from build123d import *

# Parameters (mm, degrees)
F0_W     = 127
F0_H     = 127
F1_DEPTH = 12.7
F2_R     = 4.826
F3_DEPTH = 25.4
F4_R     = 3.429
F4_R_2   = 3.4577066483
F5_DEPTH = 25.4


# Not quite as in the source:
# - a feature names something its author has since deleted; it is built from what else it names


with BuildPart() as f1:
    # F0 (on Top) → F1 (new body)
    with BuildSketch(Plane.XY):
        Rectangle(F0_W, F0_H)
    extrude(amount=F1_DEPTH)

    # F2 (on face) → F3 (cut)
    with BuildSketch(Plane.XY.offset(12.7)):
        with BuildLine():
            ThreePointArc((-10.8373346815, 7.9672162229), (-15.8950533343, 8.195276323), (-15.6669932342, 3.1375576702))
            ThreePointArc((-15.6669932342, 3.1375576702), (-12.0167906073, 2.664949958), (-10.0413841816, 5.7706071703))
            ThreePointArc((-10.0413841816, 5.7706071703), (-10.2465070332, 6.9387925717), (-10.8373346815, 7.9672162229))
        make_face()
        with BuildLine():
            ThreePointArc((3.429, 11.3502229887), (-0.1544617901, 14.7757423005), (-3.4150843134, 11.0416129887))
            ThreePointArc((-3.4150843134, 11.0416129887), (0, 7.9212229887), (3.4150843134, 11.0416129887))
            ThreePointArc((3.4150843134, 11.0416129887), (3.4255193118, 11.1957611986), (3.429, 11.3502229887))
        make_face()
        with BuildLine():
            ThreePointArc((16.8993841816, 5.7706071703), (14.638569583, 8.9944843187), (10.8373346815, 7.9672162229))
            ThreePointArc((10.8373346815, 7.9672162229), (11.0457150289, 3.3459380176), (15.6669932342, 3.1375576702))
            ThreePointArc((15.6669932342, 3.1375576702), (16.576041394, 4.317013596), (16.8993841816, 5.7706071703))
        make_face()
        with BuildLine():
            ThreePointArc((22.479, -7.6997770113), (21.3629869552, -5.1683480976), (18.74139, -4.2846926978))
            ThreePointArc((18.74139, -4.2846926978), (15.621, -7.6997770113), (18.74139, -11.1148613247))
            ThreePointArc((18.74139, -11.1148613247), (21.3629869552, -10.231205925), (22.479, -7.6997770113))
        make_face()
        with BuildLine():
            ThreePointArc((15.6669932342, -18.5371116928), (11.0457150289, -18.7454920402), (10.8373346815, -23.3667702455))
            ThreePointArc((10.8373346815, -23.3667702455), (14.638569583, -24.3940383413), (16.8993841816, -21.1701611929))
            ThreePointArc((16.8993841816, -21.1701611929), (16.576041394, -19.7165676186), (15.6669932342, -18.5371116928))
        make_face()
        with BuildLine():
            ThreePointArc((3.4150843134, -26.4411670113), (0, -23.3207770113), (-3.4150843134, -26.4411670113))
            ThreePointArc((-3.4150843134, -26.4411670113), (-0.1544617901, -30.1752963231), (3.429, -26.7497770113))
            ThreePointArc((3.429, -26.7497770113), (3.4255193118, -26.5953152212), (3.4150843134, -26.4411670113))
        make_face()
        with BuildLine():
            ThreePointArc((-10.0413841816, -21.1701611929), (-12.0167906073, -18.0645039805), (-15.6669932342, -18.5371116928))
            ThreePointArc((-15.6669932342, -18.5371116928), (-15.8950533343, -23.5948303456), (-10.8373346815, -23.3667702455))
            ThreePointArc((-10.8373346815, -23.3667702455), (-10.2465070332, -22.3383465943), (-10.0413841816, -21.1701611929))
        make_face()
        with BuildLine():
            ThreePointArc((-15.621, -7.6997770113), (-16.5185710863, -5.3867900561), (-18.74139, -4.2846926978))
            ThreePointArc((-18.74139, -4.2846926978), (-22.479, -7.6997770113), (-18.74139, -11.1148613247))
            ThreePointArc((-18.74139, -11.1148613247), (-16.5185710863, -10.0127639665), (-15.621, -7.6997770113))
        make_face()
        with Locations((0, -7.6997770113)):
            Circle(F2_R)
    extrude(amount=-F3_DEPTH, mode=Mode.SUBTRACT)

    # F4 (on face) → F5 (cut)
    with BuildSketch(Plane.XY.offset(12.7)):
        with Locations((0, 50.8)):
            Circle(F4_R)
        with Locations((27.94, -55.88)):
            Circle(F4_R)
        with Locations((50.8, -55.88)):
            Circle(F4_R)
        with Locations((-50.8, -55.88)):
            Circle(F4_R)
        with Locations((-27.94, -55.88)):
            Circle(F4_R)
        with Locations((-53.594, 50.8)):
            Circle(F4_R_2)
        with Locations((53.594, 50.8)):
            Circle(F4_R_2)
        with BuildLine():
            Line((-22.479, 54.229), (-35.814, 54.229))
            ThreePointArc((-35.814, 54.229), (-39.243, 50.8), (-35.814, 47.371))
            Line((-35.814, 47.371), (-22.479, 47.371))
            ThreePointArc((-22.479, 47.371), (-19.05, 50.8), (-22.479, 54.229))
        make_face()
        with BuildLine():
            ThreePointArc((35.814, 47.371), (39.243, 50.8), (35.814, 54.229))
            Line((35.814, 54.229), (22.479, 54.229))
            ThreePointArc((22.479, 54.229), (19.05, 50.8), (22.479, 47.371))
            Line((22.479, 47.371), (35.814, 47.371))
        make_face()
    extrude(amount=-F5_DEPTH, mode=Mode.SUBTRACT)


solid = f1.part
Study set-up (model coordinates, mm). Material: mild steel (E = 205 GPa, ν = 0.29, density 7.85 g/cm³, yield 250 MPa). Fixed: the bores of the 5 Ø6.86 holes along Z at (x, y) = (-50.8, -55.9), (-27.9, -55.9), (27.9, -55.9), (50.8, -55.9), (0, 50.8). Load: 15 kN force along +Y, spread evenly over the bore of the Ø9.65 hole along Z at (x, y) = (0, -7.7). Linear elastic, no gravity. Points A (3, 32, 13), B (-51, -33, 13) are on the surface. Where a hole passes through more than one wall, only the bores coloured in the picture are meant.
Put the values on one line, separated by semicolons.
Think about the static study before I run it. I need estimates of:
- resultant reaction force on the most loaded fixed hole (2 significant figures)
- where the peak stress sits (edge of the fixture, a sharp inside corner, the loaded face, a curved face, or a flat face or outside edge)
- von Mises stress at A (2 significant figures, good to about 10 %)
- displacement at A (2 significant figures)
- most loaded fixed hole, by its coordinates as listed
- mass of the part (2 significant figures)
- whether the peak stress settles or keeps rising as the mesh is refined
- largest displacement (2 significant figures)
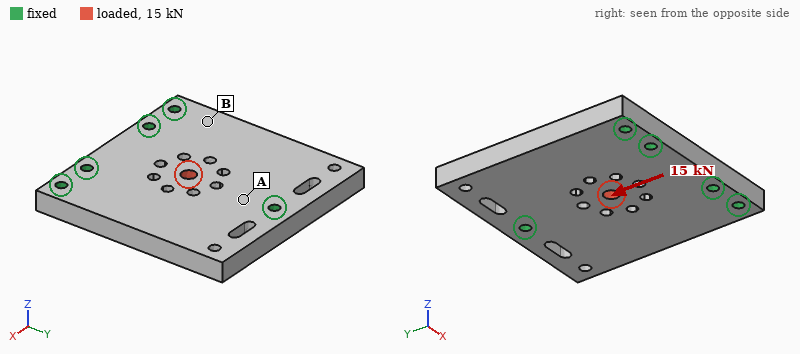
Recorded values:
4.7 kN; a sharp inside corner; 14 MPa; 1.3 µm; (0, 50.8); 1.5 kg; keeps rising; 5.4 µm
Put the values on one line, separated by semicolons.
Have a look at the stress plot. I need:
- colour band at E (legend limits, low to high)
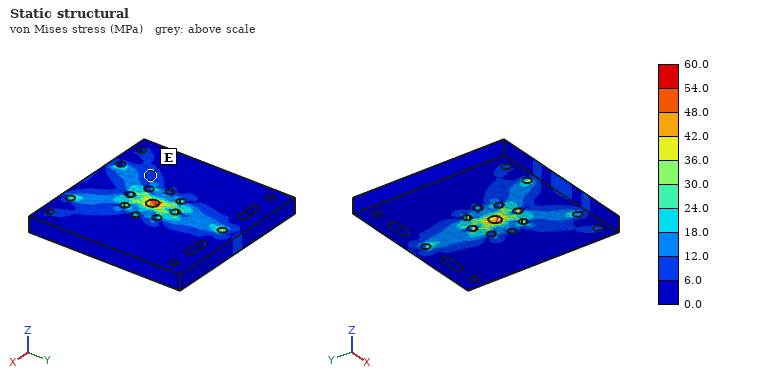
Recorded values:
6.0 to 12.0 MPa
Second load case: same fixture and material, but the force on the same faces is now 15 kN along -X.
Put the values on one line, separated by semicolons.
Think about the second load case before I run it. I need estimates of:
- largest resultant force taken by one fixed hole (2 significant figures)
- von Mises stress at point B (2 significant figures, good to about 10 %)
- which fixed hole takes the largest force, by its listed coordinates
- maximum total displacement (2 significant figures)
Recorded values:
5.1 kN; 7.7 MPa; (0, 50.8); 7.2 µm
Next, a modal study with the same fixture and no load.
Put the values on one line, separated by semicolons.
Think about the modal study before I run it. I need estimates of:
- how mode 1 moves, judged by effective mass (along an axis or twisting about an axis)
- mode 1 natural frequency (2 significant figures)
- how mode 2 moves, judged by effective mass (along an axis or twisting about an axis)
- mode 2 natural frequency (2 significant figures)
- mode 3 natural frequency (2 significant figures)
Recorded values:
twisting about Y; 2600 Hz; along Z; 3000 Hz; 5000 Hz
